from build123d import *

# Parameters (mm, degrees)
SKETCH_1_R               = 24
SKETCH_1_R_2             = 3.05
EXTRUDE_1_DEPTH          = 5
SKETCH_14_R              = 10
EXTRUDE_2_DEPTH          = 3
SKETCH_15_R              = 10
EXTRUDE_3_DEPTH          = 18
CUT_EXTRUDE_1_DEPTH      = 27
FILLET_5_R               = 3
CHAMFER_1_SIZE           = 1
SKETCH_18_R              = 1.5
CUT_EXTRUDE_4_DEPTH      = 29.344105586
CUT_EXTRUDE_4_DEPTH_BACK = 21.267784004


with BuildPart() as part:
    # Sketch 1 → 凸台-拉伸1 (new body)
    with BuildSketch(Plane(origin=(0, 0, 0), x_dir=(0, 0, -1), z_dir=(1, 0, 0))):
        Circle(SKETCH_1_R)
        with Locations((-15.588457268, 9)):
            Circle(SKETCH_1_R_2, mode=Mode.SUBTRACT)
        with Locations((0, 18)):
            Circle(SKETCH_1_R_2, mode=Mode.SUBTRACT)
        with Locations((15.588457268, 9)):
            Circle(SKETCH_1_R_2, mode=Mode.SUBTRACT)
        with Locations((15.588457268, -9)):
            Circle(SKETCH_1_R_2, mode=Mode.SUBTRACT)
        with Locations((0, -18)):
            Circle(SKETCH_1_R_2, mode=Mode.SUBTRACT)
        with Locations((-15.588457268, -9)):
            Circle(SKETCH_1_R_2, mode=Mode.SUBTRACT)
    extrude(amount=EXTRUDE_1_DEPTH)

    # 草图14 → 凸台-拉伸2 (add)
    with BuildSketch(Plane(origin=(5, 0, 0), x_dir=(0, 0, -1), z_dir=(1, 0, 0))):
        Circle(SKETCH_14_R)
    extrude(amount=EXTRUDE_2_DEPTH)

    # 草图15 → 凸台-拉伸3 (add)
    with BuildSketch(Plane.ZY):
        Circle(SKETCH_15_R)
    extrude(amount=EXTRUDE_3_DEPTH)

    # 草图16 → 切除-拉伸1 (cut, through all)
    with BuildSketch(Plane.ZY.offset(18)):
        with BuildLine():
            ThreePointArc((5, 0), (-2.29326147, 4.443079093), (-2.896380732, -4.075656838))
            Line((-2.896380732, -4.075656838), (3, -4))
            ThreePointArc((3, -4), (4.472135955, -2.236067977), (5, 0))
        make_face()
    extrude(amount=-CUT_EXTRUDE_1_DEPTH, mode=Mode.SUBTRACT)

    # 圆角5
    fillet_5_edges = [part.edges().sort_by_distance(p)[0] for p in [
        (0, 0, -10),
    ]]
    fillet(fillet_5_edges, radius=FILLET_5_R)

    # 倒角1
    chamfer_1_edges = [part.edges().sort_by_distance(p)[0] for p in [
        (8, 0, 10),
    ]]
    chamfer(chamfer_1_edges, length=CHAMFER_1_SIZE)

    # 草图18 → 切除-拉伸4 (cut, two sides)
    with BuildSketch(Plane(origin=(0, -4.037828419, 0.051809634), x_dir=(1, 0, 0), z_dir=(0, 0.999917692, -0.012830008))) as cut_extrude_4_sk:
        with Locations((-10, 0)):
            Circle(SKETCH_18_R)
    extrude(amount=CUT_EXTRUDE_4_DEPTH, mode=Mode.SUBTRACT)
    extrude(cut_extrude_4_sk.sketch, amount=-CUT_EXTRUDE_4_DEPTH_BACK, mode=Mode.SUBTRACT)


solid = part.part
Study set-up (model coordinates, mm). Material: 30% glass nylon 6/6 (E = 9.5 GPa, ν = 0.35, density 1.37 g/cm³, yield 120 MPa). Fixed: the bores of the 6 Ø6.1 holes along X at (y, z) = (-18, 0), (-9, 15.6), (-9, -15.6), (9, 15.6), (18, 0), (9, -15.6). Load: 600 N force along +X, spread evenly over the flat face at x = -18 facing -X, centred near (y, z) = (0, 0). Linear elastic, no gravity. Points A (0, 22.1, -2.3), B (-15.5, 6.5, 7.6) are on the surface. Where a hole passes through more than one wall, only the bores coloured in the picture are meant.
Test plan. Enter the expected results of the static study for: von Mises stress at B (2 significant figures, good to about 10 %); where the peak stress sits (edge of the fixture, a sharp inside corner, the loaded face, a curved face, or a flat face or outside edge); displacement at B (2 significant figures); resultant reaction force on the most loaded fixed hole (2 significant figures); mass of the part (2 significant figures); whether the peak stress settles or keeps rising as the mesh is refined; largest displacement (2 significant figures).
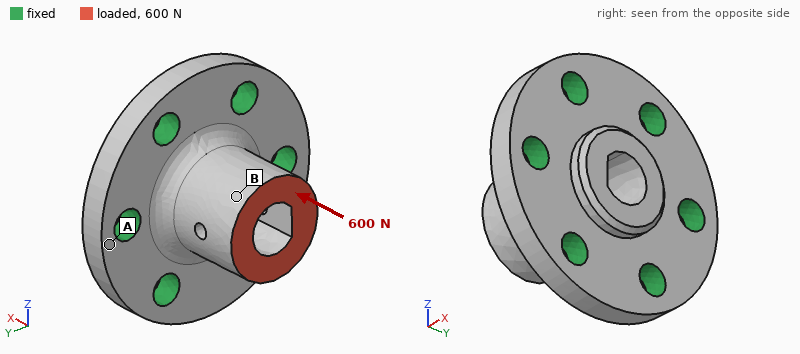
2.5 MPa
edge of the fixture
9.6 µm
110 N
18 g
keeps rising
11 µm
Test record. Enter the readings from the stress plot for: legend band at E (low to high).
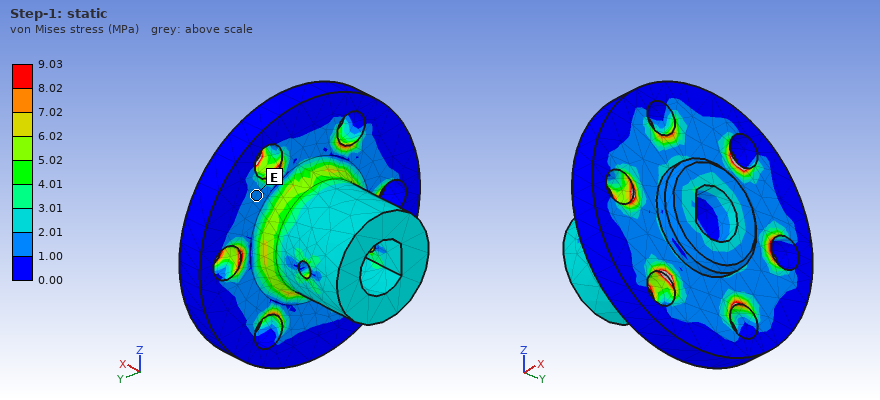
1.00 to 2.01 MPa
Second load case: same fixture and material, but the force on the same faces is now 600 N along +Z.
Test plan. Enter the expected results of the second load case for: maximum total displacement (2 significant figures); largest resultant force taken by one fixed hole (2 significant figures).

69 µm
290 N
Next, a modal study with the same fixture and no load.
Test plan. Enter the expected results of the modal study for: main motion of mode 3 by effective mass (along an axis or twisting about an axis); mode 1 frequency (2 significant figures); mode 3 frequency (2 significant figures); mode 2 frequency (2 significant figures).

along X
11 kHz
16 kHz
11 kHz
